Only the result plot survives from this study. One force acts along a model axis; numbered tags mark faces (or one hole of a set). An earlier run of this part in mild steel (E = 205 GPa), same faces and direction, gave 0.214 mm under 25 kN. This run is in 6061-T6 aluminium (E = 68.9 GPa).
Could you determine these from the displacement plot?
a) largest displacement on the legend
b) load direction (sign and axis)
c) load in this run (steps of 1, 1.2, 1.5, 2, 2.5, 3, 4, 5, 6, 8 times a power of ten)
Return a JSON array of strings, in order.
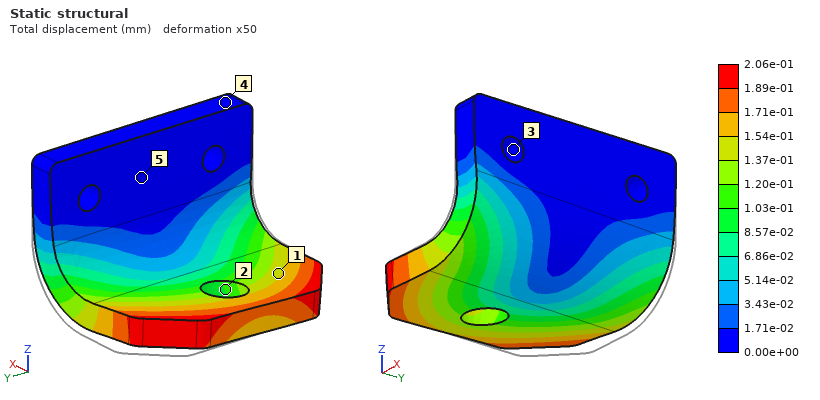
["2.06e-01 mm", "-Y", "8 kN"]
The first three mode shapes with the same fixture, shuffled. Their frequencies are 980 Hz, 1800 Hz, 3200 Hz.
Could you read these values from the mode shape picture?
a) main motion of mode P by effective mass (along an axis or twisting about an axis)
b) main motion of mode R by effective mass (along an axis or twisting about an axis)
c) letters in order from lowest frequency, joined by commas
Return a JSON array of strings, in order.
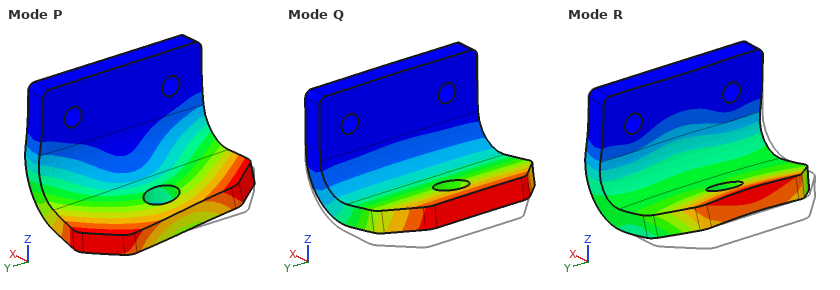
["along Y", "along X", "Q, P, R"]
